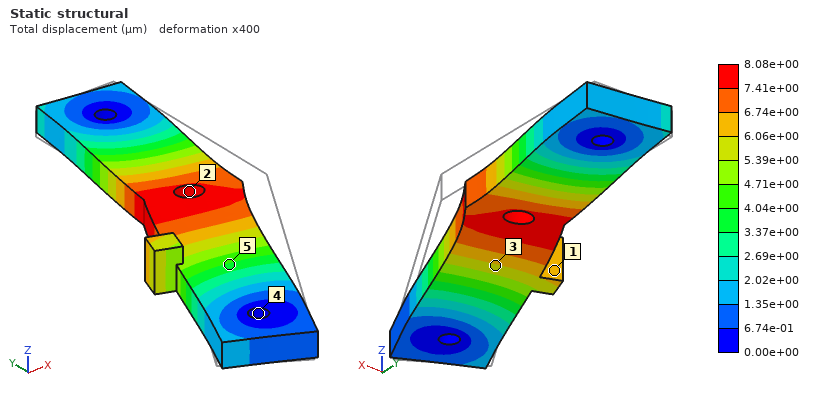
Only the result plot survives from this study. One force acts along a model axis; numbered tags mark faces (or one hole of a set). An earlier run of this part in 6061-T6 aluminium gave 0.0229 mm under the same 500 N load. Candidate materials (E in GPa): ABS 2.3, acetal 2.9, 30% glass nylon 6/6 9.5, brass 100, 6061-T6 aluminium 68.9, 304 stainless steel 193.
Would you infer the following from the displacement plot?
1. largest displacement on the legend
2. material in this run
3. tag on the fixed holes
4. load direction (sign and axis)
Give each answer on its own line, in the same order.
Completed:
8.08e+00 µm
304 stainless steel
4
-X
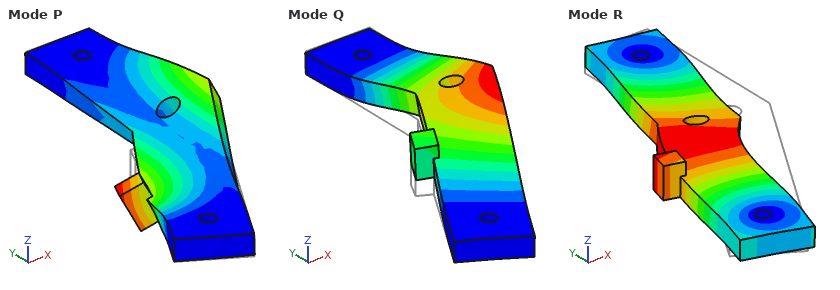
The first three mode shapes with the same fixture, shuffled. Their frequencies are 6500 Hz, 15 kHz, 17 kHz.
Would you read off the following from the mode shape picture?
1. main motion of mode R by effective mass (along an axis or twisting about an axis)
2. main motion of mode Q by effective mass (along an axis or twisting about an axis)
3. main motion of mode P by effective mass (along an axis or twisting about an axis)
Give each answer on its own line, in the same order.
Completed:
along X
along Z
twisting about Y
